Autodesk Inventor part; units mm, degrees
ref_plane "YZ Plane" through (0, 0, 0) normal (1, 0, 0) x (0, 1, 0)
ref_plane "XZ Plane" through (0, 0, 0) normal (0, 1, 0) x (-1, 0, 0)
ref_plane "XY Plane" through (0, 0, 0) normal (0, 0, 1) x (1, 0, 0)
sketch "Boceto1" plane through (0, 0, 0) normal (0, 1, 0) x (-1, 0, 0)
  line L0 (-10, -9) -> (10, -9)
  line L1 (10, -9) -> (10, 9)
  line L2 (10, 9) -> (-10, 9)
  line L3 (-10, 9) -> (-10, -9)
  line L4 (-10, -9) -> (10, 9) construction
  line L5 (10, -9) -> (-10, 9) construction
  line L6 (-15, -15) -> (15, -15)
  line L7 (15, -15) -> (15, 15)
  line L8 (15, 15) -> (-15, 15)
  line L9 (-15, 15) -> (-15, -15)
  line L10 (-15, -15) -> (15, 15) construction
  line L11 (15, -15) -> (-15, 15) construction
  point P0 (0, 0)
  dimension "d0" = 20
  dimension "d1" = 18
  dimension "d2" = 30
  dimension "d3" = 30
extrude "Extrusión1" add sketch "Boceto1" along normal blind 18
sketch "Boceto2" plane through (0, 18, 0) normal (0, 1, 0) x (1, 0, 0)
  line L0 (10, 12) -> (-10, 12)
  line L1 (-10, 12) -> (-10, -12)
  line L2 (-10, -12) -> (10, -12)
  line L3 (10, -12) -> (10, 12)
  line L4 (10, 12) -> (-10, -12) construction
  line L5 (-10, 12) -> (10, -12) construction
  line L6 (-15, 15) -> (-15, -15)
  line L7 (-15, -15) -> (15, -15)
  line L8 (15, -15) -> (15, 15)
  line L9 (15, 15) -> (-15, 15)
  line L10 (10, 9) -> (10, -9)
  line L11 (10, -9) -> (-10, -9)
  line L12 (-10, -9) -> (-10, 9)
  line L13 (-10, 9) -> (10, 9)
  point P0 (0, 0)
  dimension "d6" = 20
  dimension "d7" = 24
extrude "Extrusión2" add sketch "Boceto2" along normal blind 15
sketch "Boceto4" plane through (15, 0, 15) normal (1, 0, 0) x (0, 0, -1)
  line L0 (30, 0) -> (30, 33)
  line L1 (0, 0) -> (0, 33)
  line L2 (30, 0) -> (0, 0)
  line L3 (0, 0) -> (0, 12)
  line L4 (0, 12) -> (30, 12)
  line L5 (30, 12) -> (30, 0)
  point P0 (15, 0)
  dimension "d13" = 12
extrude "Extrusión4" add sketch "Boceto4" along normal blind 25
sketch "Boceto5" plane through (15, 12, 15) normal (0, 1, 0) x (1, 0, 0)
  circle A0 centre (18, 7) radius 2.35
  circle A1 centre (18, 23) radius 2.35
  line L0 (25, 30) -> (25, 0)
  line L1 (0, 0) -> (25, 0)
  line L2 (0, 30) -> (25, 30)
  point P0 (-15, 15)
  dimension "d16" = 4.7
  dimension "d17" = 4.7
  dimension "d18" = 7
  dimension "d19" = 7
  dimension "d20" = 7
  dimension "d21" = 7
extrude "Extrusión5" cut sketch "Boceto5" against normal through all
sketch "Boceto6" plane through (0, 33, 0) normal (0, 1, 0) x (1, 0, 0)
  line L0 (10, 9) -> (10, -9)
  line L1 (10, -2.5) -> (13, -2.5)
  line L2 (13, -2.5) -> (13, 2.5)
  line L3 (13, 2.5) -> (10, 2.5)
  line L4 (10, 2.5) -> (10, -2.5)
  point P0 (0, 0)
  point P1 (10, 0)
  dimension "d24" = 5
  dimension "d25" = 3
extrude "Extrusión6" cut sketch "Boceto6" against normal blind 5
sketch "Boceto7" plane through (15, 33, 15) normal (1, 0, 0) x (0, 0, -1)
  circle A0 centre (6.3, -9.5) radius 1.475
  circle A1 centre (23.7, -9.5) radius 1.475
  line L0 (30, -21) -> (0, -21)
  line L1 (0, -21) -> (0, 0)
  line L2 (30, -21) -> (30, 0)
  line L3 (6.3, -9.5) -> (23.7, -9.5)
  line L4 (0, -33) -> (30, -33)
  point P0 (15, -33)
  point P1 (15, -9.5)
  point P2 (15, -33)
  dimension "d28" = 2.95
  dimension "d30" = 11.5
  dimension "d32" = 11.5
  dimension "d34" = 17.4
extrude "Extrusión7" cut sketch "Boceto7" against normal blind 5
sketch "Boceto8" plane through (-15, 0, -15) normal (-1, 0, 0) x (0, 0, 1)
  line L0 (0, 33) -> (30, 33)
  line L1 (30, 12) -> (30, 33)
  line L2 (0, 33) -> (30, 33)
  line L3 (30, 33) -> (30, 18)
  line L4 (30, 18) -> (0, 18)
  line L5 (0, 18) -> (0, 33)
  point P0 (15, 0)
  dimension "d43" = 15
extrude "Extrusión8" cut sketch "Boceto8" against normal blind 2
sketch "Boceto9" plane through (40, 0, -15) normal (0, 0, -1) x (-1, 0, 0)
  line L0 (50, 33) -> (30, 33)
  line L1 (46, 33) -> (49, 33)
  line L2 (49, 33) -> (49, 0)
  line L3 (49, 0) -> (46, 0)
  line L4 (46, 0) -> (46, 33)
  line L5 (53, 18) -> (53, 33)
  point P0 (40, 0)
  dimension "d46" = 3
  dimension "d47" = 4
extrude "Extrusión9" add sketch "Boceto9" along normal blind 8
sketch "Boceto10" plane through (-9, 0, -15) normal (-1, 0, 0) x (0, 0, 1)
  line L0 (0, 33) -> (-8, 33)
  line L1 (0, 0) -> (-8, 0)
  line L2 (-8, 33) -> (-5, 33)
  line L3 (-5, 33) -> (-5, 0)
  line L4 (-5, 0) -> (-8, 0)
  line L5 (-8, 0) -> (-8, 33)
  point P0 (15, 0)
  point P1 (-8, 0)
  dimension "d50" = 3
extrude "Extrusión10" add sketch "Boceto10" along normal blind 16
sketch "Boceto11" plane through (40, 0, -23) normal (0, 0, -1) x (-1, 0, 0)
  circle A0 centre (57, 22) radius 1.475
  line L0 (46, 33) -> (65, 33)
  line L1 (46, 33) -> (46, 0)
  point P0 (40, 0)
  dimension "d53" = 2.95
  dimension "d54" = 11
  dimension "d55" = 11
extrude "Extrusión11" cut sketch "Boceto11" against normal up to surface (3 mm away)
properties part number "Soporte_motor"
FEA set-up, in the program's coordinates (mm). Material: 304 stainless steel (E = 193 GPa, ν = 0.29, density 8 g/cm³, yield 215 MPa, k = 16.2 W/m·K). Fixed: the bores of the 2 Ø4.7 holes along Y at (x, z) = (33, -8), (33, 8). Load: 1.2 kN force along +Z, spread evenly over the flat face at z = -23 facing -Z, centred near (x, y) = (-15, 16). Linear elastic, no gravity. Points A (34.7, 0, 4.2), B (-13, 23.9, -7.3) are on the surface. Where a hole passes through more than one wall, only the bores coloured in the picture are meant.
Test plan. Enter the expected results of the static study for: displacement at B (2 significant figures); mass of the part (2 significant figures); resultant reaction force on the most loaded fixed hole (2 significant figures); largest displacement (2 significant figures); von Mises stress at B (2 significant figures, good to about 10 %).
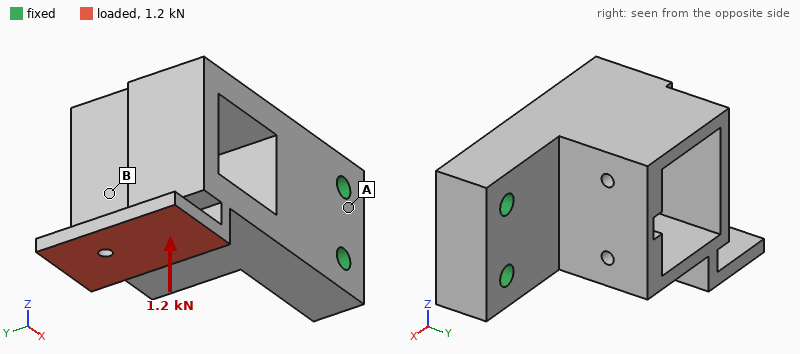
0.037 mm
210 g
3.1 kN
0.18 mm
39 MPa
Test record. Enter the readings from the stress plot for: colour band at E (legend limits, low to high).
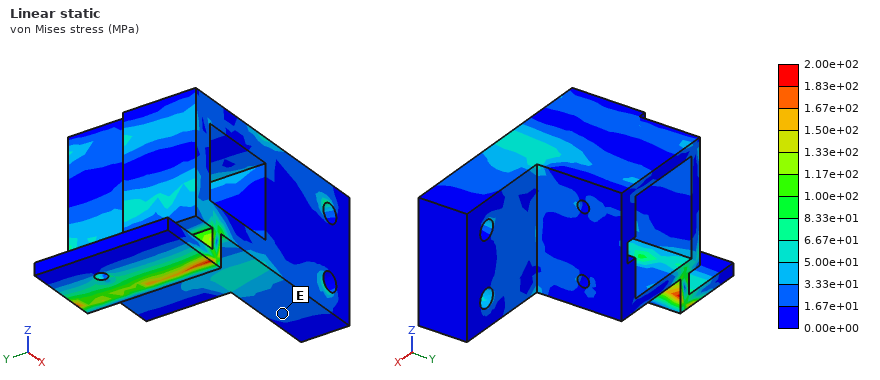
1.67e+01 to 3.33e+01 MPa
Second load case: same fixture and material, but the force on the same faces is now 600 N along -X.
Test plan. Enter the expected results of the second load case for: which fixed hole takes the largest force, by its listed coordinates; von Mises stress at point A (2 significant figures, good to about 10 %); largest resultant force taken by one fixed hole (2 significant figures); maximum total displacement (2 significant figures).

(33, -8)
3.5 MPa
1.0 kN
52 µm
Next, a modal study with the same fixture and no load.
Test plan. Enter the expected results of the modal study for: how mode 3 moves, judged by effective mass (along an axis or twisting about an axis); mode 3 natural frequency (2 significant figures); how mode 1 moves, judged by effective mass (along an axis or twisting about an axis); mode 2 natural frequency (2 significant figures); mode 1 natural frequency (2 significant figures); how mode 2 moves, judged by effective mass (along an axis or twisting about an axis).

twisting about X
4800 Hz
along Y
3300 Hz
2500 Hz
along Z
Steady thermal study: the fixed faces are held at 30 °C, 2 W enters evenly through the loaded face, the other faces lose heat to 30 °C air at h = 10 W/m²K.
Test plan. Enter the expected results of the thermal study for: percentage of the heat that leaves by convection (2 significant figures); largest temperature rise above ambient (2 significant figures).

44 %
29 K
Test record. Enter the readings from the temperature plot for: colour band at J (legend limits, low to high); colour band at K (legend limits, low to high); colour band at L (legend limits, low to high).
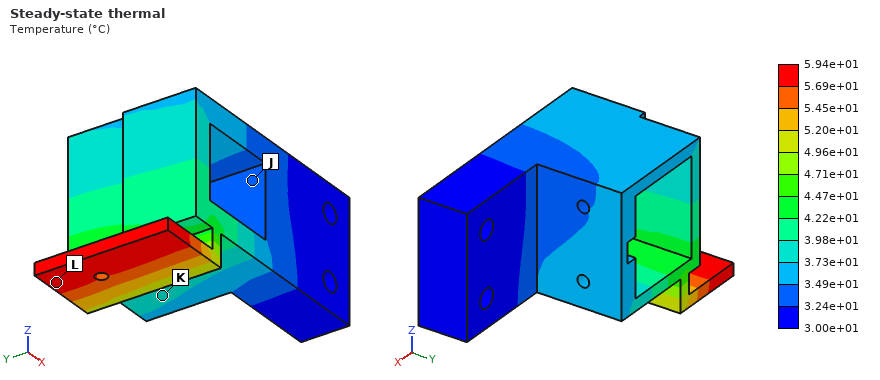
3.24e+01 to 3.49e+01 °C
3.73e+01 to 3.98e+01 °C
5.69e+01 to 5.94e+01 °C
